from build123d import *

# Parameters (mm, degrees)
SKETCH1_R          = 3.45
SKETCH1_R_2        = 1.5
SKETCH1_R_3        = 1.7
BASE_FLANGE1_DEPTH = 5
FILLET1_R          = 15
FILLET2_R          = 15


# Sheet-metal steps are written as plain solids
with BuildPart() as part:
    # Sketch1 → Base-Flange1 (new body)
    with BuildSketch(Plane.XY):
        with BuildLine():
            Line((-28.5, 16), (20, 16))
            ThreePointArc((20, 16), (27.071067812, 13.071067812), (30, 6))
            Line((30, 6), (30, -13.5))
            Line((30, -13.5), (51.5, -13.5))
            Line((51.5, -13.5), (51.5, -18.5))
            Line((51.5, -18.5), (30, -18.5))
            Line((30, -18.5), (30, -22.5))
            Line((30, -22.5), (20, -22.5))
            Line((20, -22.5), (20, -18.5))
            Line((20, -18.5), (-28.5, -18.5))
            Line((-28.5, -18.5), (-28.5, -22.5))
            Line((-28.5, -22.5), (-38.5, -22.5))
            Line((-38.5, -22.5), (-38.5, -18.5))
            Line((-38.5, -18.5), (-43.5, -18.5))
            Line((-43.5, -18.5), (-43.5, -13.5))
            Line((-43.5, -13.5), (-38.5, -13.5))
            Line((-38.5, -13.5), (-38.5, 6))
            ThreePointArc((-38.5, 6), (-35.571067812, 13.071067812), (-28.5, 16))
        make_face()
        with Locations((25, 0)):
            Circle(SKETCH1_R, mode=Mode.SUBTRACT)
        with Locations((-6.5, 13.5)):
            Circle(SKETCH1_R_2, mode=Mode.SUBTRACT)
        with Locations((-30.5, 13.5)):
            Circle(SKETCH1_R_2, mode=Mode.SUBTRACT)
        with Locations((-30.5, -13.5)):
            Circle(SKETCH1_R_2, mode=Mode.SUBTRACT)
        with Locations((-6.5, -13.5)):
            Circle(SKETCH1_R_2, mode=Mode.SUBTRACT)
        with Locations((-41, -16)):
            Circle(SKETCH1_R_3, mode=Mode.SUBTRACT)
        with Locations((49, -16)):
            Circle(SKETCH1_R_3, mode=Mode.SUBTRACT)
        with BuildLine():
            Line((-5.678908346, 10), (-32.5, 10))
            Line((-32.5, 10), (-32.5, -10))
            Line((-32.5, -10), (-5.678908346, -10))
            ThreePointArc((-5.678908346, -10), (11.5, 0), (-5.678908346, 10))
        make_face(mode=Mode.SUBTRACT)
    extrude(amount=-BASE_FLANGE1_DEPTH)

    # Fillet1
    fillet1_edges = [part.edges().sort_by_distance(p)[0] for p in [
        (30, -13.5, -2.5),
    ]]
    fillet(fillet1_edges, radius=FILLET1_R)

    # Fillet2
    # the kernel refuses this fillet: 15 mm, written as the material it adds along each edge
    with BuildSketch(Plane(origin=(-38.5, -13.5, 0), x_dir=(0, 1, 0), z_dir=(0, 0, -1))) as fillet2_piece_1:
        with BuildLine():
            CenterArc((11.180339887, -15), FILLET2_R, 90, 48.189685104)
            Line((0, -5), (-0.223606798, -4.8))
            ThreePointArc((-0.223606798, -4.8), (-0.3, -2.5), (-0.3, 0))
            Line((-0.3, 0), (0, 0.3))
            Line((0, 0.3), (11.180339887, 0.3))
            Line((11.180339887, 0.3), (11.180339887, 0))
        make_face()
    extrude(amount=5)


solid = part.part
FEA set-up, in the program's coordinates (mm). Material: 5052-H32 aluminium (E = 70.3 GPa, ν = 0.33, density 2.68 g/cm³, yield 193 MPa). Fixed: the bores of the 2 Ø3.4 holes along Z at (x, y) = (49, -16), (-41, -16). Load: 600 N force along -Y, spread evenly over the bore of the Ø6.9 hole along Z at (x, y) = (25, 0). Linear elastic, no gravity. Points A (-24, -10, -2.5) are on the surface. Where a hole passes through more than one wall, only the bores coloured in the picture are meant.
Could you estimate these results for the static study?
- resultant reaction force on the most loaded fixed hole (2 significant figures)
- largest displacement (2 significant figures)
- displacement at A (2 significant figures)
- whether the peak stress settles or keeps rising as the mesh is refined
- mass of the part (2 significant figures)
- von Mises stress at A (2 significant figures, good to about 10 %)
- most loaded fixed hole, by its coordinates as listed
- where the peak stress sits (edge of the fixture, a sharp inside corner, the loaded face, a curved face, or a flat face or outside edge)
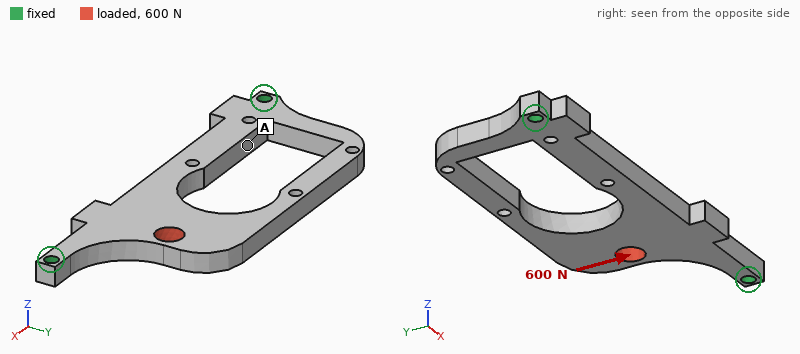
530 N
55 µm
14 µm
keeps rising
22 g
15 MPa
(49, -16)
edge of the fixture
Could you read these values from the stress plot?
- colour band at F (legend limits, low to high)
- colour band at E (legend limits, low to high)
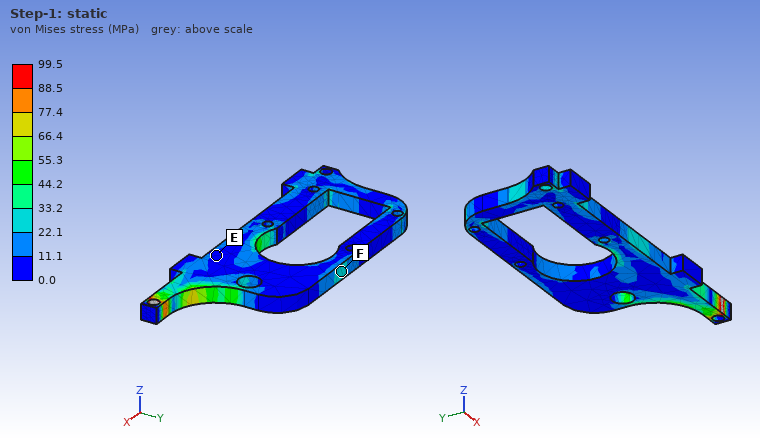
22.1 to 33.2 MPa
0.0 to 11.1 MPa
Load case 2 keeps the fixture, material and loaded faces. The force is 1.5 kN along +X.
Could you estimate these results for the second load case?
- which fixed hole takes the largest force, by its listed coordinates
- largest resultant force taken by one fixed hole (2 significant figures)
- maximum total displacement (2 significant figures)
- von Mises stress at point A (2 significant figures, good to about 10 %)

(49, -16)
870 N
90 µm
23 MPa
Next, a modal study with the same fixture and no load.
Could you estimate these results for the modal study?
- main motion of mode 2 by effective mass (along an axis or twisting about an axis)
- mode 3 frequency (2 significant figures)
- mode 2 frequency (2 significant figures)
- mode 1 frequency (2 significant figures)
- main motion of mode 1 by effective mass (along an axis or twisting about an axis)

along Z
4000 Hz
3400 Hz
1400 Hz
along Z
